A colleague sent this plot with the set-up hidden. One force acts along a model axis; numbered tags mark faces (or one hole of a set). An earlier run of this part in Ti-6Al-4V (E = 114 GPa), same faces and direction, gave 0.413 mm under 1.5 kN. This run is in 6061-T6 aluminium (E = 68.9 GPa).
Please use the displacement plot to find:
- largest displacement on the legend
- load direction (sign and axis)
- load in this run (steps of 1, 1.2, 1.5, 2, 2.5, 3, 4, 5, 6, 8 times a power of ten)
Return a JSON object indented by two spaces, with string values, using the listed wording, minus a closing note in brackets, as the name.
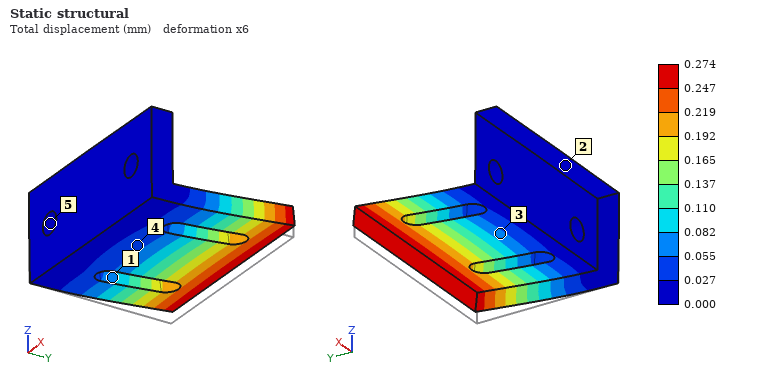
{
  "largest displacement on the legend": "0.274 mm",
  "load direction": "+Z",
  "load in this run": "600 N"
}
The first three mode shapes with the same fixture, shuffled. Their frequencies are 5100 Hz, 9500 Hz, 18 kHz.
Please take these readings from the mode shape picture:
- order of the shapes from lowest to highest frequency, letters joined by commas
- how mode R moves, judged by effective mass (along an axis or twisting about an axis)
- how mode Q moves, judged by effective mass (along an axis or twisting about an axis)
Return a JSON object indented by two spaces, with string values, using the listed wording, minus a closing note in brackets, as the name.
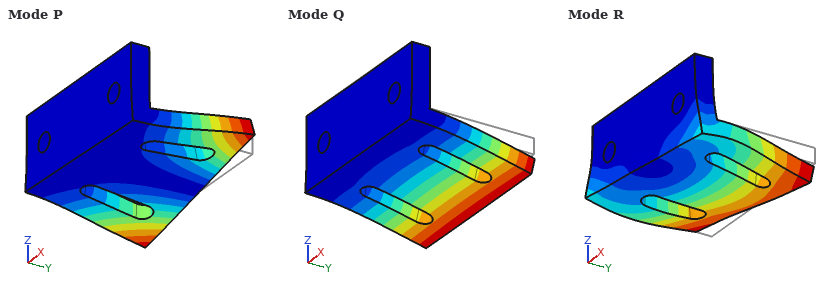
{
  "order of the shapes from lowest to highest frequency, letters joined by commas": "Q, P, R",
  "how mode R moves, judged by effective mass": "along X",
  "how mode Q moves, judged by effective mass": "along Z"
}
